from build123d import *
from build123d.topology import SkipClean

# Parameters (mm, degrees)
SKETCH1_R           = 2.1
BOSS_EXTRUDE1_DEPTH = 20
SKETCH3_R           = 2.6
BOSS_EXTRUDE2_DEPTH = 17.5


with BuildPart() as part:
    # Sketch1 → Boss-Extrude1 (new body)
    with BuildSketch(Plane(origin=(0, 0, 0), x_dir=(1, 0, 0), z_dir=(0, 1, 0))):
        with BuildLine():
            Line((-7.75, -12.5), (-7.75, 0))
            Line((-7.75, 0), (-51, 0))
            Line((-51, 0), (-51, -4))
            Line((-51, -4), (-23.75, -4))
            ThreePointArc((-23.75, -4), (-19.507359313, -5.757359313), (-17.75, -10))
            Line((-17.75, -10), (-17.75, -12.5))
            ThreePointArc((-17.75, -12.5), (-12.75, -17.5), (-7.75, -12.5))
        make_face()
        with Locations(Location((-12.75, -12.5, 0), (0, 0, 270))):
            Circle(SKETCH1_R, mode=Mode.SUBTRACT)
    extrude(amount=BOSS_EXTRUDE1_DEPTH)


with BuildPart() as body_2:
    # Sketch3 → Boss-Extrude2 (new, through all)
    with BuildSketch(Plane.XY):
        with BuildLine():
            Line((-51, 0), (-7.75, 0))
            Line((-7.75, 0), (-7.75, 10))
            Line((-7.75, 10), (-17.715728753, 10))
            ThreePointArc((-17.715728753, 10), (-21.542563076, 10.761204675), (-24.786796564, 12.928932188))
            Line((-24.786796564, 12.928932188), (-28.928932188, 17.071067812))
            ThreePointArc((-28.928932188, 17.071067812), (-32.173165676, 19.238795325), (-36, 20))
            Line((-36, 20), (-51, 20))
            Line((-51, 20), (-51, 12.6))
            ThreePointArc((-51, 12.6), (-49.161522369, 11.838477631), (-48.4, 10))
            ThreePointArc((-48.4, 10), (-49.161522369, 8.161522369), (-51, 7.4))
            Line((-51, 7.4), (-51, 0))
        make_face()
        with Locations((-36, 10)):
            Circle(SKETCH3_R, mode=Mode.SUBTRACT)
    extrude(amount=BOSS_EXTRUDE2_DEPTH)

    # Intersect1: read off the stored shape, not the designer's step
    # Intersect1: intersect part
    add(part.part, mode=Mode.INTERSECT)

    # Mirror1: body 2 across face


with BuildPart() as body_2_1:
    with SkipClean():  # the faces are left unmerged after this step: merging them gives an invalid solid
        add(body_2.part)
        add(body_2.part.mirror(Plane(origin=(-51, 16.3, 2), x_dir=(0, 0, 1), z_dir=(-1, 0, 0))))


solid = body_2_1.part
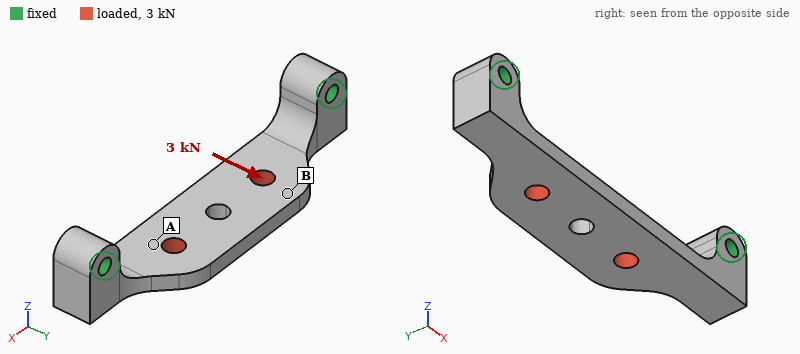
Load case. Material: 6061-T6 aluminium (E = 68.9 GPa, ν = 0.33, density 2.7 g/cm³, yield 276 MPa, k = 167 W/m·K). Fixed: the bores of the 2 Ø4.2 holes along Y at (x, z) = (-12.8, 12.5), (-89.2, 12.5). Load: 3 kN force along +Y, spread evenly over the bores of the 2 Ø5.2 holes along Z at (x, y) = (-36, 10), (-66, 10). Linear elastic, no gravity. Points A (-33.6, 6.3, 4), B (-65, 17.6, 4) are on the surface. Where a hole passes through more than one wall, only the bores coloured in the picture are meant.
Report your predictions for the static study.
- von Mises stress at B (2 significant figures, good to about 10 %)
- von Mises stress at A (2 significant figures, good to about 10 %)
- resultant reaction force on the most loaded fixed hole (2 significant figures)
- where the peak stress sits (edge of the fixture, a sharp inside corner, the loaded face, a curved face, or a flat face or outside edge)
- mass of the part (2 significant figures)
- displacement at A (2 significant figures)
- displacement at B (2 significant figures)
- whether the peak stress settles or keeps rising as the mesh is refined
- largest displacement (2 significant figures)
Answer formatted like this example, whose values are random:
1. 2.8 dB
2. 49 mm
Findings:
1. 69 MPa
2. 31 MPa
3. 1.6 kN
4. edge of the fixture
5. 20 g
6. 0.083 mm
7. 0.094 mm
8. keeps rising
9. 0.11 mm
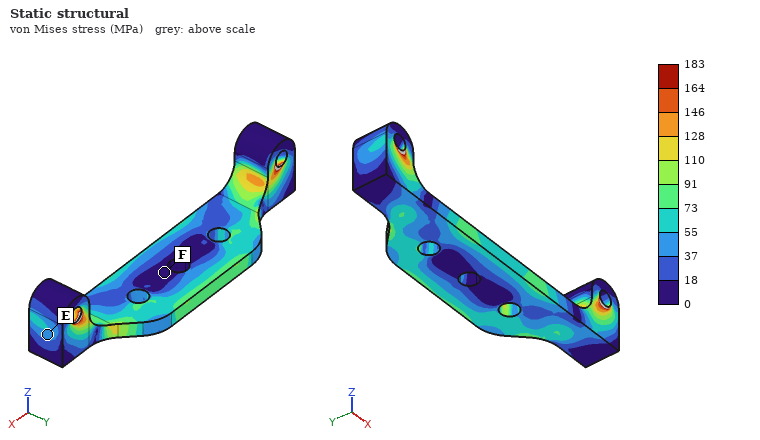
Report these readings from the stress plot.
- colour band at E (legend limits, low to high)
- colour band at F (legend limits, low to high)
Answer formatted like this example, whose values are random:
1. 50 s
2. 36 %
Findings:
1. 37 to 55 MPa
2. 0 to 18 MPa
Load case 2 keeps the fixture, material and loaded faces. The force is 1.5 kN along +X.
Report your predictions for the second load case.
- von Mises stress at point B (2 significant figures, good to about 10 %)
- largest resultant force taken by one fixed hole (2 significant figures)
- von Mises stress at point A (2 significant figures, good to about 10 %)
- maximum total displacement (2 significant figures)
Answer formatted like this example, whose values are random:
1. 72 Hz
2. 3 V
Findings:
1. 7.2 MPa
2. 760 N
3. 27 MPa
4. 20 µm
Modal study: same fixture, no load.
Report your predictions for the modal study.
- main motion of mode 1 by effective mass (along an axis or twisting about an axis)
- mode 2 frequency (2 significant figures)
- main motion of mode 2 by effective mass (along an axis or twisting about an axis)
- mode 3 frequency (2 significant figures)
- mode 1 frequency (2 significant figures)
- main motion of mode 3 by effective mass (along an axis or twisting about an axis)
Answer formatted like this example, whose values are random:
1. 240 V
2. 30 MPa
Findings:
1. along Z
2. 7700 Hz
3. twisting about X
4. 8900 Hz
5. 3900 Hz
6. along Y
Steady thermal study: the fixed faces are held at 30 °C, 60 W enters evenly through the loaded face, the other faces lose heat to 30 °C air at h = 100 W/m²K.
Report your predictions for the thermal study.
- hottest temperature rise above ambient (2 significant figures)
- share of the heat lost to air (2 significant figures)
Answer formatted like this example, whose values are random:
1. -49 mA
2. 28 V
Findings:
1. 68 K
2. 25 %
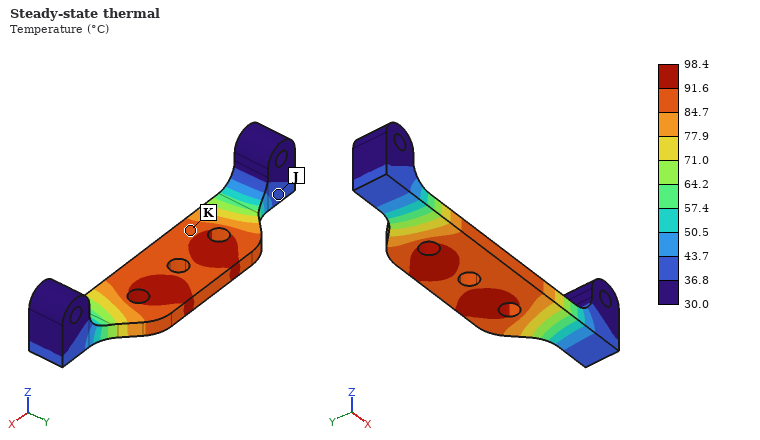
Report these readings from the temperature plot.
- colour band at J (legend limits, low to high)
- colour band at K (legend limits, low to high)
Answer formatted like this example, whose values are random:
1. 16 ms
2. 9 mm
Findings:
1. 36.8 to 43.7 °C
2. 84.7 to 91.6 °C
